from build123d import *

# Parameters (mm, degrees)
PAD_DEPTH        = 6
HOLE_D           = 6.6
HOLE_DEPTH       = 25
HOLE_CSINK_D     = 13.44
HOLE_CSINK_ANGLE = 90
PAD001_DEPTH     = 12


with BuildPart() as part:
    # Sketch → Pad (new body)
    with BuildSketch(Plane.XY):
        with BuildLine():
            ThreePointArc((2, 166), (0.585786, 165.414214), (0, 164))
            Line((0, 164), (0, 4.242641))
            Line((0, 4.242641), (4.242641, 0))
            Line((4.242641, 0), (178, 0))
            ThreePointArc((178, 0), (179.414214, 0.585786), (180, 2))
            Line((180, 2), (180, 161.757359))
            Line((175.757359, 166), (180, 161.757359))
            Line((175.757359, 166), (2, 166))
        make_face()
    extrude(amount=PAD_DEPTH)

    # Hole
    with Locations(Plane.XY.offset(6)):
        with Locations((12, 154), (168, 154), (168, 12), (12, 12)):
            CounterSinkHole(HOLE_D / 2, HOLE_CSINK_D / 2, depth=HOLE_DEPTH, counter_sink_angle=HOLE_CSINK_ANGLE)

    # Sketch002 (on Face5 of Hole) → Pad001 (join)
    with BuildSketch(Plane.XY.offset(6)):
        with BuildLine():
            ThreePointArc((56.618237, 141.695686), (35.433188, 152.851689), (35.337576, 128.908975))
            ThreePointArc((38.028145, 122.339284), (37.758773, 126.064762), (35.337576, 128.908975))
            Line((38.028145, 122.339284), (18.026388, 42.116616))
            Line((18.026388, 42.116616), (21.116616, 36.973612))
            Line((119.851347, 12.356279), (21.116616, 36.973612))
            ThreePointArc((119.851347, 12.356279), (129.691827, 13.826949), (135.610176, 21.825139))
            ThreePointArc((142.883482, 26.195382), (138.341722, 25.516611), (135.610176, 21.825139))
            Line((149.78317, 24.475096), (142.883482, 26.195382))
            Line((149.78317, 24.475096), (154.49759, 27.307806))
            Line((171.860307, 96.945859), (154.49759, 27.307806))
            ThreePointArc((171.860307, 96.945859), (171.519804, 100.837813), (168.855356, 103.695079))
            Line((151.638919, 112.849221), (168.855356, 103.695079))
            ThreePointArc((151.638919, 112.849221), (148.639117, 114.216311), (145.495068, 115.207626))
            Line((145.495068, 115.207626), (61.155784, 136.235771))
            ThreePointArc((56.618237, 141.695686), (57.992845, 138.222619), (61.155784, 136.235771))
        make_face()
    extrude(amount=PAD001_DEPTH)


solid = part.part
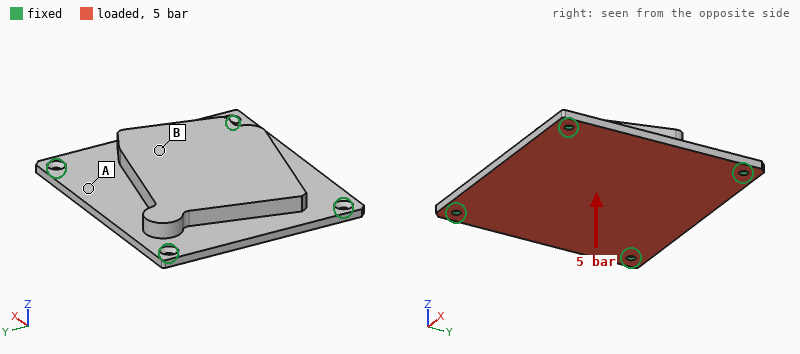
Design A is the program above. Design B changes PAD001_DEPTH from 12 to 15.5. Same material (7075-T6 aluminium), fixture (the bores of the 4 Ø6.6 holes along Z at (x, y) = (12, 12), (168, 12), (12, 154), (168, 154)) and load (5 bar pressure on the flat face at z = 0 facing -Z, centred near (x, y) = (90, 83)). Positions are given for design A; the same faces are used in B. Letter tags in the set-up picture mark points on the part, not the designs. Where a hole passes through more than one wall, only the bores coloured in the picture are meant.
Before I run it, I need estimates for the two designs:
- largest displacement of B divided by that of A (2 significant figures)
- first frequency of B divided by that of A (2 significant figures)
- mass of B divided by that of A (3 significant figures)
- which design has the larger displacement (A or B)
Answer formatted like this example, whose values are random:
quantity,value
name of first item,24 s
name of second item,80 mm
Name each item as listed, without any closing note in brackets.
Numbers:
quantity,value
largest displacement of B divided by that of A,0.89
first frequency of B divided by that of A,0.99
mass of B divided by that of A,1.14
which design has the larger displacement,A
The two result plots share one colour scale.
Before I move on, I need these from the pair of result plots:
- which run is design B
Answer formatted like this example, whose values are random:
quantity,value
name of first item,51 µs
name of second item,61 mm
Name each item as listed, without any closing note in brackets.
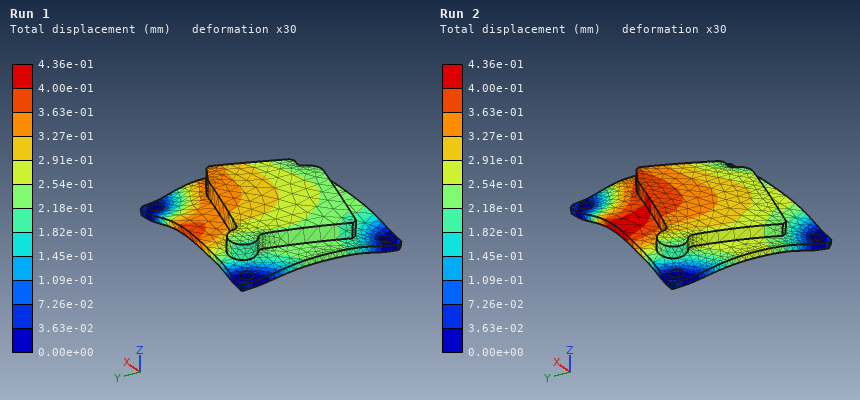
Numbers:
quantity,value
which run is design B,Run 1
